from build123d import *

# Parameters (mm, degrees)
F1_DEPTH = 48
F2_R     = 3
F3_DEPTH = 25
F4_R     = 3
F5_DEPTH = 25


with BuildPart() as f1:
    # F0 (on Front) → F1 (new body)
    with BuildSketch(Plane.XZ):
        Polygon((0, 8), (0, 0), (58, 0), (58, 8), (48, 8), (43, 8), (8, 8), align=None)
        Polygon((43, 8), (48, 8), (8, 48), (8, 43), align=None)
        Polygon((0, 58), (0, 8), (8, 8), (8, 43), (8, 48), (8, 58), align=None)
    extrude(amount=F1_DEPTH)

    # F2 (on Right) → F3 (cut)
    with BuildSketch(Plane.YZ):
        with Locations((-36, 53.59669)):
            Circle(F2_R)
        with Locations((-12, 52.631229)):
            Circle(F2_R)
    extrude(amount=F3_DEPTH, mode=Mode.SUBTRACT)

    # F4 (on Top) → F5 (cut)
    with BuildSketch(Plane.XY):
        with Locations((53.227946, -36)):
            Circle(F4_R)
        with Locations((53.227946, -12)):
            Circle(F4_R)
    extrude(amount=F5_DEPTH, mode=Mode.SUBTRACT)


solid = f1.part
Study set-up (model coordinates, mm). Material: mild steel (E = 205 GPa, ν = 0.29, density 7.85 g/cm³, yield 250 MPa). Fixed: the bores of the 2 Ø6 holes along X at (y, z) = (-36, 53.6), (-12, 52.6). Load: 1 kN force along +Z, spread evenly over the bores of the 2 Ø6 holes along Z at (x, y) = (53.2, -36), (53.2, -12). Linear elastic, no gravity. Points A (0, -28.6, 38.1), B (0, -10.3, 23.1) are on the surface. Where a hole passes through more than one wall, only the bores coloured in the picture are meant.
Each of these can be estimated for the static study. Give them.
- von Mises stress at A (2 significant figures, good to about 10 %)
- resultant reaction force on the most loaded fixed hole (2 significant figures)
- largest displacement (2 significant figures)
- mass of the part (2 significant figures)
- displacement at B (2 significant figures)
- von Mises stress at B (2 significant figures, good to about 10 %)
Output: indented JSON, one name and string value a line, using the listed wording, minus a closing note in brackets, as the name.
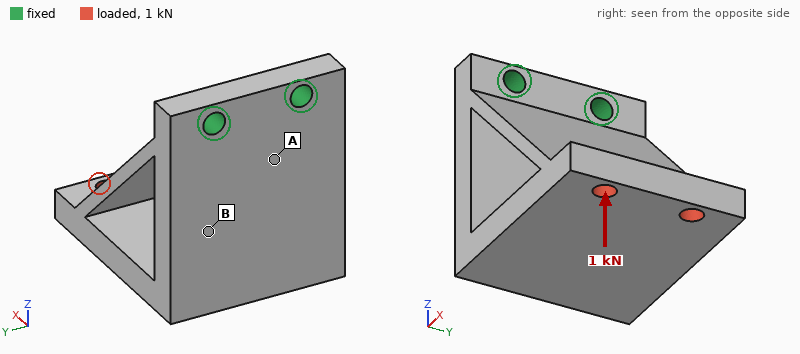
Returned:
{
  "von Mises stress at A": "55 MPa",
  "resultant reaction force on the most loaded fixed hole": "510 N",
  "largest displacement": "0.14 mm",
  "mass of the part": "390 g",
  "displacement at B": "0.041 mm",
  "von Mises stress at B": "24 MPa"
}
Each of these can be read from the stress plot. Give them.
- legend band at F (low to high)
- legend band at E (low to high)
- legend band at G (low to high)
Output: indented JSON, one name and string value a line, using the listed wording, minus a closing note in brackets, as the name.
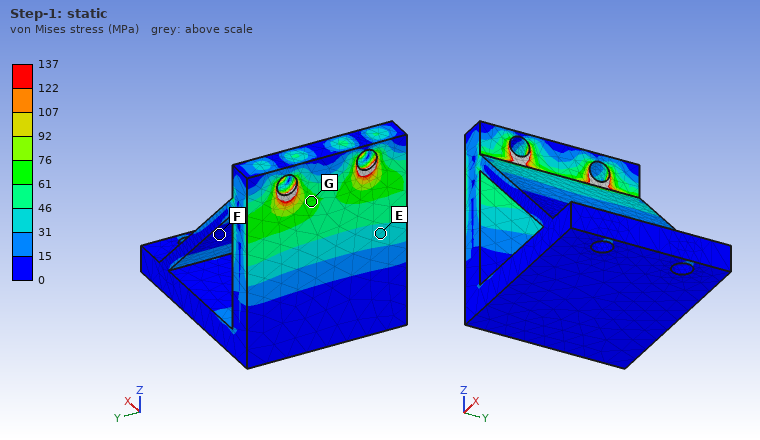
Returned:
{
  "legend band at F": "0 to 15 MPa",
  "legend band at E": "31 to 46 MPa",
  "legend band at G": "61 to 76 MPa"
}
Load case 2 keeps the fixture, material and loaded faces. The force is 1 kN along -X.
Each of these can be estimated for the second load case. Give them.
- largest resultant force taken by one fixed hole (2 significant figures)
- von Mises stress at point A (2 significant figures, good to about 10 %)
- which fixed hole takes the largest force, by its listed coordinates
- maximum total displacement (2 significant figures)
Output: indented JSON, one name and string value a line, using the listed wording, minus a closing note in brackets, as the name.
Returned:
{
  "largest resultant force taken by one fixed hole": "560 N",
  "von Mises stress at point A": "50 MPa",
  "which fixed hole takes the largest force, by its listed coordinates": "(-12, 52.6)",
  "maximum total displacement": "0.13 mm"
}
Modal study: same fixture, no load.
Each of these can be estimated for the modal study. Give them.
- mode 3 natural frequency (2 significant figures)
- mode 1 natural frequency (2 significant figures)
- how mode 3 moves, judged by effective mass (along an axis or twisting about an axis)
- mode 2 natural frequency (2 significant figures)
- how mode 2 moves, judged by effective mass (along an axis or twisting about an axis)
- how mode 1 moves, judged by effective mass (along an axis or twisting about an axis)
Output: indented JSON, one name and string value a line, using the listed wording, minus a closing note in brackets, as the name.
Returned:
{
  "mode 3 natural frequency": "5600 Hz",
  "mode 1 natural frequency": "1000 Hz",
  "how mode 3 moves, judged by effective mass": "along Y",
  "mode 2 natural frequency": "3200 Hz",
  "how mode 2 moves, judged by effective mass": "along Y",
  "how mode 1 moves, judged by effective mass": "along X"
}
